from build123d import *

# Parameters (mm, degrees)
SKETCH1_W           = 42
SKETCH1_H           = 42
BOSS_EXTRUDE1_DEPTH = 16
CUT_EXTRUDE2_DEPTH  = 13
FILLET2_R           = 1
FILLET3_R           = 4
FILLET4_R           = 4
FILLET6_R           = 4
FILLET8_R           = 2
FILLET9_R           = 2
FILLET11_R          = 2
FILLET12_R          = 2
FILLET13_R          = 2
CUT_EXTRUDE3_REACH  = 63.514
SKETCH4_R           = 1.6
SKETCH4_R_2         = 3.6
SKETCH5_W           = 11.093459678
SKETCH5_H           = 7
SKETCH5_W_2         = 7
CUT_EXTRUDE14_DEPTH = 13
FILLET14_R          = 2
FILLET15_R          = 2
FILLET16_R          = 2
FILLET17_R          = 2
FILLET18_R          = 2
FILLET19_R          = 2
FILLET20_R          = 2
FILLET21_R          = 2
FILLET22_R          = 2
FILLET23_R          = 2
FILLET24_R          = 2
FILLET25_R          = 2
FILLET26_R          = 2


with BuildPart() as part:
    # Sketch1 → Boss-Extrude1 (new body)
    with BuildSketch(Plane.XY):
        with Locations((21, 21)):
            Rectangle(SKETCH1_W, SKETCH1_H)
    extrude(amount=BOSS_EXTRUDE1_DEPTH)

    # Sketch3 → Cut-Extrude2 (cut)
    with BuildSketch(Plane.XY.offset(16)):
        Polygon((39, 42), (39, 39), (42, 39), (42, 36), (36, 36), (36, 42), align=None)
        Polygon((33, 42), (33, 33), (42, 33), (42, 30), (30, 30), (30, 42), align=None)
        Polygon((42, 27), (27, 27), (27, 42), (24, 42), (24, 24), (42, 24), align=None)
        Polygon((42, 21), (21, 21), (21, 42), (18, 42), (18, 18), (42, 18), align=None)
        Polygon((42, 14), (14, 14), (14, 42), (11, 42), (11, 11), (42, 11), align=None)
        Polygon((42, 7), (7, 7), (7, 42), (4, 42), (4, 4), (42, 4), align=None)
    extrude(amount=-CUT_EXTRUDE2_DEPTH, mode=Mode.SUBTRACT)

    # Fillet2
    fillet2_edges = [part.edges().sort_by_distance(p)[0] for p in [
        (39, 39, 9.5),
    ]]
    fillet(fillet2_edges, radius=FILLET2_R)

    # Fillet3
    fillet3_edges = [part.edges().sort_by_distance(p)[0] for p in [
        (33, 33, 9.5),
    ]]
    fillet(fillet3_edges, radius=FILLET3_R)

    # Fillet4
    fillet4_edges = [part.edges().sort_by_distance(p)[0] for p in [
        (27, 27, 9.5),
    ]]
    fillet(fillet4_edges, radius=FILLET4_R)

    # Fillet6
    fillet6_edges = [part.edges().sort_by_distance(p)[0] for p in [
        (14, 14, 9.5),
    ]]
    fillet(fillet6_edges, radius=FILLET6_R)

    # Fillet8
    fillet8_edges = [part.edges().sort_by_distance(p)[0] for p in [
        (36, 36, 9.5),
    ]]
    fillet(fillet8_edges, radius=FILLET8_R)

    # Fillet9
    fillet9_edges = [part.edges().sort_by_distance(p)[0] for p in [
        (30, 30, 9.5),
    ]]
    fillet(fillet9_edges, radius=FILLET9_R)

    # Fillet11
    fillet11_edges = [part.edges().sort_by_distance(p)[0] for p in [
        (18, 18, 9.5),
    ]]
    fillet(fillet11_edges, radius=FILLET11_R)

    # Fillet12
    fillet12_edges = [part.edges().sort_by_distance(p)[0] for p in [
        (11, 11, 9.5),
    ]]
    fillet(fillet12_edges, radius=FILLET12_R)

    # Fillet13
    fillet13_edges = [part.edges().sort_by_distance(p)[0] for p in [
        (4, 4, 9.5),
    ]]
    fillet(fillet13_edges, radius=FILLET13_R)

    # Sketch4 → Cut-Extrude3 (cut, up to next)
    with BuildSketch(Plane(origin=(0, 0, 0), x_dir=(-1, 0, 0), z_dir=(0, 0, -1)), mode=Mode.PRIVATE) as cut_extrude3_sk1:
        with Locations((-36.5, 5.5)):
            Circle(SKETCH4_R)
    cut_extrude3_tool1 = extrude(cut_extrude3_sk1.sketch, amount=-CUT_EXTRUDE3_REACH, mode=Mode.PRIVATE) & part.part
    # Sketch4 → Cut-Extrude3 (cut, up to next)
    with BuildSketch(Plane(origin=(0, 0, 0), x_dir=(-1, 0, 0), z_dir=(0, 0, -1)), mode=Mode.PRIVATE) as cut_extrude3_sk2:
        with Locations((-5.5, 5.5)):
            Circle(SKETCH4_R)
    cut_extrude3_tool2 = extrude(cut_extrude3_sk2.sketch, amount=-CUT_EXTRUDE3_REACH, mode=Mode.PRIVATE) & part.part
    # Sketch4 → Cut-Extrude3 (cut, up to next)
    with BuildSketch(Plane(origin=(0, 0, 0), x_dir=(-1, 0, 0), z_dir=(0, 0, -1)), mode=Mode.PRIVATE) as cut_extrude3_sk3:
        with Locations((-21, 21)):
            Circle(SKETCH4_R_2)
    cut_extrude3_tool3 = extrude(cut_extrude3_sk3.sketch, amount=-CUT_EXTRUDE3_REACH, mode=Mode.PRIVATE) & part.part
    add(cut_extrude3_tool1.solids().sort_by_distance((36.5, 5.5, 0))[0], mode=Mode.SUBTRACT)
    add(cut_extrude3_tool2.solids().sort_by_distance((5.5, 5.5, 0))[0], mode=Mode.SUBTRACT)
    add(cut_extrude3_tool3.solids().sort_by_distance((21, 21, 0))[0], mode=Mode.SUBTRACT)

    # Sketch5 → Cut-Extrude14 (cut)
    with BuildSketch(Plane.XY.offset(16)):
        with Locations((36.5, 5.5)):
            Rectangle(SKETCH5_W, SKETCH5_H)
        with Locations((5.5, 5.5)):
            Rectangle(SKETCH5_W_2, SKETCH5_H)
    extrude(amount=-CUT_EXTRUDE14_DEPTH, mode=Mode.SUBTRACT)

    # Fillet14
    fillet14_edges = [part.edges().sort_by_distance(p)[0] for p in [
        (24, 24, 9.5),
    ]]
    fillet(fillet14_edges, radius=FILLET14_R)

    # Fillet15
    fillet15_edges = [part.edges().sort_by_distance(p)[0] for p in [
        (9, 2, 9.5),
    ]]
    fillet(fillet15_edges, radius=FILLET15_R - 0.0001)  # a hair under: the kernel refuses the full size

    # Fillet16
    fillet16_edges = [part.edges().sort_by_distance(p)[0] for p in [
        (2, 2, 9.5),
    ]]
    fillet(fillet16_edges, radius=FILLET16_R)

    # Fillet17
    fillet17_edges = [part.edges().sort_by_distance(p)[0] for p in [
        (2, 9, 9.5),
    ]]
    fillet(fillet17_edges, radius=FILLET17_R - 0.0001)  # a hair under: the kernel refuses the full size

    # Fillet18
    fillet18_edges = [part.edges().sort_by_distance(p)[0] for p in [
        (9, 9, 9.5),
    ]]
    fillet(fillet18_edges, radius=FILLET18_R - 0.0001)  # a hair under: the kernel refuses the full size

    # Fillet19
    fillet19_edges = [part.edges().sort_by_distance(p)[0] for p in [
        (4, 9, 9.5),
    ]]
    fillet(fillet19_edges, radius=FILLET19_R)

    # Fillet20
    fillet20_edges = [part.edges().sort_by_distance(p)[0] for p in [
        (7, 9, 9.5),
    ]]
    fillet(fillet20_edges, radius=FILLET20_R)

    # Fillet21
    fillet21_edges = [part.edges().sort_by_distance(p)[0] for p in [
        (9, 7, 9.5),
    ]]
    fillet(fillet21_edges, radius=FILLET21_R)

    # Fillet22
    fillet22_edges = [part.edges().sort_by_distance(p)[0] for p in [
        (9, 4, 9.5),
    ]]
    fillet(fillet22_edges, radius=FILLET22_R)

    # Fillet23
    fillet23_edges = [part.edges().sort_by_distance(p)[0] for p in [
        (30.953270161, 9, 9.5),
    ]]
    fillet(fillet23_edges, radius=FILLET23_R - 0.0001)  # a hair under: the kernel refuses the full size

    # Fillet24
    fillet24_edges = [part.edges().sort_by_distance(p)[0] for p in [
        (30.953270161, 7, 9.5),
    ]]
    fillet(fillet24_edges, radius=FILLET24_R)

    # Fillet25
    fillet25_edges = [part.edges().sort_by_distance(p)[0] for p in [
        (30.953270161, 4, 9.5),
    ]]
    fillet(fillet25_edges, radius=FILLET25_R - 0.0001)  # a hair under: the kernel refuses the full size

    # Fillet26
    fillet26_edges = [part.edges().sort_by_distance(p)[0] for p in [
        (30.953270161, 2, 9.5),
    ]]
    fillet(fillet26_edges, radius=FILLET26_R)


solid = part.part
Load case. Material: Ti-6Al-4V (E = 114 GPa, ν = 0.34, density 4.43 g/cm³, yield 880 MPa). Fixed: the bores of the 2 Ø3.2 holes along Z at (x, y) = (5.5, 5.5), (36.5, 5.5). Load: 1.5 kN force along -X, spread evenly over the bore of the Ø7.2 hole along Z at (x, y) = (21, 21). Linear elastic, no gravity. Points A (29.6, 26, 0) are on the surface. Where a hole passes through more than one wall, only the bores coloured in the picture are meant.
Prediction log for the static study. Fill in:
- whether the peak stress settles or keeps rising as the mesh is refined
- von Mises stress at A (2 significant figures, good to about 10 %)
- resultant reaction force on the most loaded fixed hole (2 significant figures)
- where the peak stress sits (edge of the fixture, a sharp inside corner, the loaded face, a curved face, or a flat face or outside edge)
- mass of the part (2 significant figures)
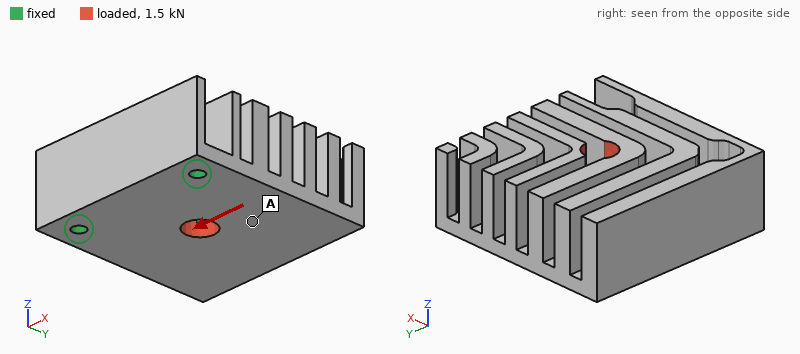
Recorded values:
keeps rising
8.3 MPa
1.1 kN
edge of the fixture
78 g
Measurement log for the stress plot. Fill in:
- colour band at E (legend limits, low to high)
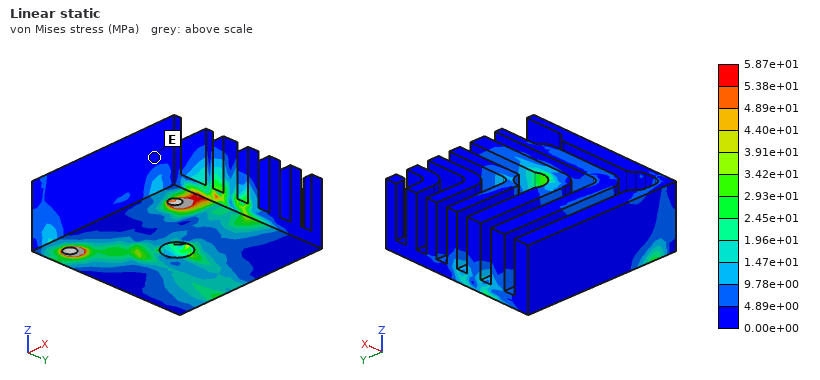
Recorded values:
0.00e+00 to 4.89e+00 MPa
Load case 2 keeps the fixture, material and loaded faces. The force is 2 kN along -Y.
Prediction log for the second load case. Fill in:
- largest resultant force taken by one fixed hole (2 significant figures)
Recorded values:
1.0 kN
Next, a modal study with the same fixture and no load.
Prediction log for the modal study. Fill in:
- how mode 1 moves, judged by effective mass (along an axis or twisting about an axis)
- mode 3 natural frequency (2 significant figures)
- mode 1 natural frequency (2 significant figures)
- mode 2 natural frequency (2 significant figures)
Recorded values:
along Z
6000 Hz
1500 Hz
3400 Hz
